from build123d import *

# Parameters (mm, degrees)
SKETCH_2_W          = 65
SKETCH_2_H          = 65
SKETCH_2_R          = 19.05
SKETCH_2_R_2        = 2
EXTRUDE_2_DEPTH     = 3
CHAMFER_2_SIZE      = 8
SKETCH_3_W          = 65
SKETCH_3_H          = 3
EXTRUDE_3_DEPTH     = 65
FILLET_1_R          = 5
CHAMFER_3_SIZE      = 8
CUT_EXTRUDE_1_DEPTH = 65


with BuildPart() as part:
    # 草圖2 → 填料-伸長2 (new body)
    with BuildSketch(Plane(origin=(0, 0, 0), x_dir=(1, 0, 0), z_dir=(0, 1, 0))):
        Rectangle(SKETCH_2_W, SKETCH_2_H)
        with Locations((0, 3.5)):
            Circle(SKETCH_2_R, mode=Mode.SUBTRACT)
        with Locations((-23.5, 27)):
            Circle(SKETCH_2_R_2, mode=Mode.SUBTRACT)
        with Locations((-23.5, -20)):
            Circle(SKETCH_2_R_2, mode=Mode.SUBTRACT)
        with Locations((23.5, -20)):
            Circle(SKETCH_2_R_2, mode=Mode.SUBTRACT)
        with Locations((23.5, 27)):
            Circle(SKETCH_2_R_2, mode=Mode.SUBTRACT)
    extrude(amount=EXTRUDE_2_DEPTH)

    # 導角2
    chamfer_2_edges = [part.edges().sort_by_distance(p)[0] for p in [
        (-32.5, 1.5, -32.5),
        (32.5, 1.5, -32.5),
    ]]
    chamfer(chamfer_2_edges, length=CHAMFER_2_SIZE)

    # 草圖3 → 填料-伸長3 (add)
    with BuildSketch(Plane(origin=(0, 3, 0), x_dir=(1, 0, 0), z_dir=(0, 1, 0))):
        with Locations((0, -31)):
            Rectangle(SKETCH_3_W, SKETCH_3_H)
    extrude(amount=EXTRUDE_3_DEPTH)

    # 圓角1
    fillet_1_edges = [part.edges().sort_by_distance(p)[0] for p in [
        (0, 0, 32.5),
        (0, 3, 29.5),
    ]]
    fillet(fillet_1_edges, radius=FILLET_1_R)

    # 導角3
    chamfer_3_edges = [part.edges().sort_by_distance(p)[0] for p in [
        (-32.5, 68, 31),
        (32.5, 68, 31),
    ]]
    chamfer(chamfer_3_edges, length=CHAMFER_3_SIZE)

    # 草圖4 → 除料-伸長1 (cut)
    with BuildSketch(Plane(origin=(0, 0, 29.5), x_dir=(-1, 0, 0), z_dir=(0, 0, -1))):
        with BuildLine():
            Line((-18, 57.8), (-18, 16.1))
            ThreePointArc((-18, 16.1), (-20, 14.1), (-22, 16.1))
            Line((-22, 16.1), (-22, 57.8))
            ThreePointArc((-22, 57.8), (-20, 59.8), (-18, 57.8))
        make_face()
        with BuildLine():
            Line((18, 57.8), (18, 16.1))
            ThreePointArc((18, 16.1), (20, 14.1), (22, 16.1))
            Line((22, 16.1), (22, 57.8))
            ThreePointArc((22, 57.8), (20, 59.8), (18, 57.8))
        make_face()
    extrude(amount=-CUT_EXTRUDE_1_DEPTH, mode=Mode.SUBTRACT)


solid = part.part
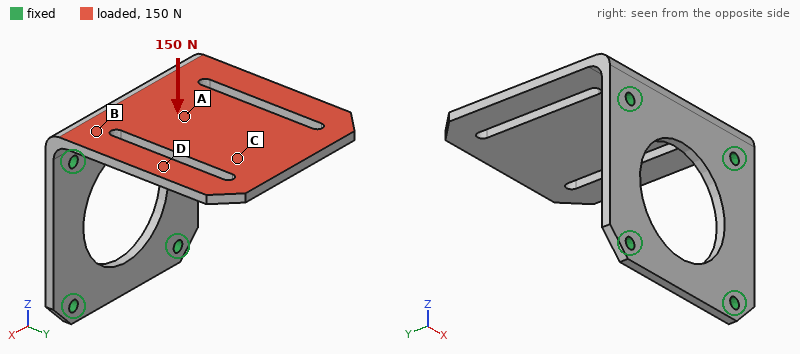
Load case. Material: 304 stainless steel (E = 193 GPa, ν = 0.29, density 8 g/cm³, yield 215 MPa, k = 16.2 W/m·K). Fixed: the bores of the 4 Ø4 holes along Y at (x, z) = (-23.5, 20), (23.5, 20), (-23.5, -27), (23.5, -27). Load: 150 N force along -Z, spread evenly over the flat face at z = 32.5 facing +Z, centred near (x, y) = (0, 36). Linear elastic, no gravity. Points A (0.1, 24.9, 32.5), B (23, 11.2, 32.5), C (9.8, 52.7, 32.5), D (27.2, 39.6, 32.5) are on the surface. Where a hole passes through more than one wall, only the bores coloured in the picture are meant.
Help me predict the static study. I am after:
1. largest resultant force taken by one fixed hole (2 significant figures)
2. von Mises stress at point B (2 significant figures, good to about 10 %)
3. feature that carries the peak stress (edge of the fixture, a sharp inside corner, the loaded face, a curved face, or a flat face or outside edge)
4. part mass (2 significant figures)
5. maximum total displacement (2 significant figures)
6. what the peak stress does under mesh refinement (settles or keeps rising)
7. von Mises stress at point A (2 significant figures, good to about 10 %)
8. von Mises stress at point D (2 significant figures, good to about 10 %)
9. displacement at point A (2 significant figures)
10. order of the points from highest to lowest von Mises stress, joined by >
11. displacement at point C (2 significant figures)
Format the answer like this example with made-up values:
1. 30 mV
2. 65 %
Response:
1. 79 N
2. 32 MPa
3. edge of the fixture
4. 160 g
5. 0.30 mm
6. keeps rising
7. 22 MPa
8. 12 MPa
9. 0.074 mm
10. B > A > D > C
11. 0.21 mm
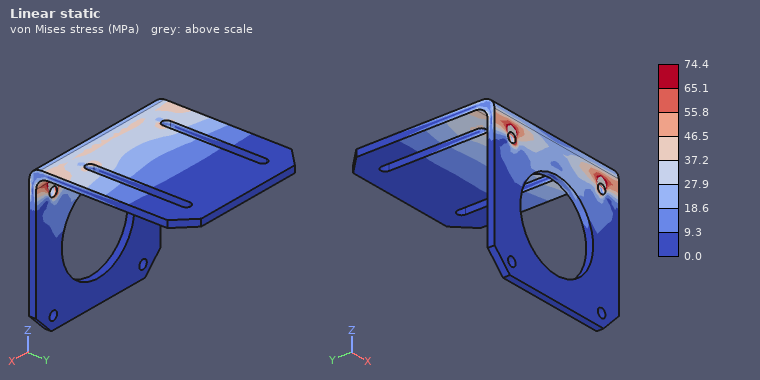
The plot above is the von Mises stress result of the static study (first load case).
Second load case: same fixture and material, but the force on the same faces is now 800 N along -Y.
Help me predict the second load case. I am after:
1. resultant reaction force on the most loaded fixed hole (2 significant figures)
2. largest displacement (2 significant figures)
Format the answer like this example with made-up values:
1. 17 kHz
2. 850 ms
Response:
1. 410 N
2. 0.22 mm
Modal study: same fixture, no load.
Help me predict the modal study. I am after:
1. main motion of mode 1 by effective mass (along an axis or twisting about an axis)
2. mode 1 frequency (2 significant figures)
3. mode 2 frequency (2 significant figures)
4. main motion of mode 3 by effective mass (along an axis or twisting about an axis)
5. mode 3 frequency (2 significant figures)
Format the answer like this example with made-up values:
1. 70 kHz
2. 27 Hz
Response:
1. along Z
2. 470 Hz
3. 1300 Hz
4. along X
5. 2500 Hz
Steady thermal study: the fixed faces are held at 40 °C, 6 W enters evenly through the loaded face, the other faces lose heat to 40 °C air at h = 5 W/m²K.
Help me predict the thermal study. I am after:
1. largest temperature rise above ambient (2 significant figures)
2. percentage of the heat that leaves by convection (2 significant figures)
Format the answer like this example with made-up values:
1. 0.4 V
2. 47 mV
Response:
1. 73 K
2. 26 %
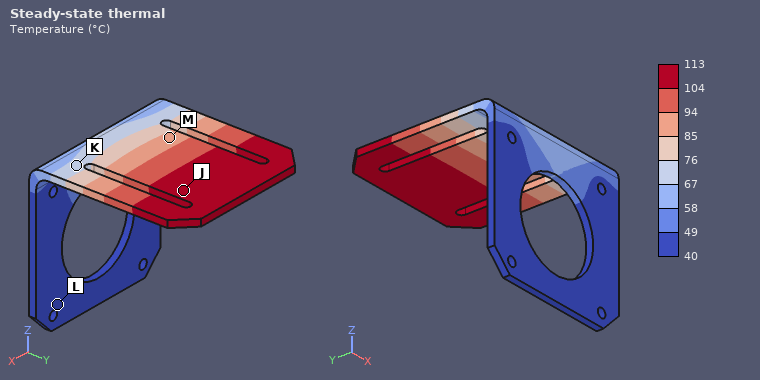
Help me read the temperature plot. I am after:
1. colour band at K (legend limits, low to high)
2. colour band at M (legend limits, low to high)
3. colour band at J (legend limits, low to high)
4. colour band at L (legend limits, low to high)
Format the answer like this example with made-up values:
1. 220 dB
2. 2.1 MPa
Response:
1. 67 to 76 °C
2. 85 to 94 °C
3. 104 to 113 °C
4. 40 to 49 °C
